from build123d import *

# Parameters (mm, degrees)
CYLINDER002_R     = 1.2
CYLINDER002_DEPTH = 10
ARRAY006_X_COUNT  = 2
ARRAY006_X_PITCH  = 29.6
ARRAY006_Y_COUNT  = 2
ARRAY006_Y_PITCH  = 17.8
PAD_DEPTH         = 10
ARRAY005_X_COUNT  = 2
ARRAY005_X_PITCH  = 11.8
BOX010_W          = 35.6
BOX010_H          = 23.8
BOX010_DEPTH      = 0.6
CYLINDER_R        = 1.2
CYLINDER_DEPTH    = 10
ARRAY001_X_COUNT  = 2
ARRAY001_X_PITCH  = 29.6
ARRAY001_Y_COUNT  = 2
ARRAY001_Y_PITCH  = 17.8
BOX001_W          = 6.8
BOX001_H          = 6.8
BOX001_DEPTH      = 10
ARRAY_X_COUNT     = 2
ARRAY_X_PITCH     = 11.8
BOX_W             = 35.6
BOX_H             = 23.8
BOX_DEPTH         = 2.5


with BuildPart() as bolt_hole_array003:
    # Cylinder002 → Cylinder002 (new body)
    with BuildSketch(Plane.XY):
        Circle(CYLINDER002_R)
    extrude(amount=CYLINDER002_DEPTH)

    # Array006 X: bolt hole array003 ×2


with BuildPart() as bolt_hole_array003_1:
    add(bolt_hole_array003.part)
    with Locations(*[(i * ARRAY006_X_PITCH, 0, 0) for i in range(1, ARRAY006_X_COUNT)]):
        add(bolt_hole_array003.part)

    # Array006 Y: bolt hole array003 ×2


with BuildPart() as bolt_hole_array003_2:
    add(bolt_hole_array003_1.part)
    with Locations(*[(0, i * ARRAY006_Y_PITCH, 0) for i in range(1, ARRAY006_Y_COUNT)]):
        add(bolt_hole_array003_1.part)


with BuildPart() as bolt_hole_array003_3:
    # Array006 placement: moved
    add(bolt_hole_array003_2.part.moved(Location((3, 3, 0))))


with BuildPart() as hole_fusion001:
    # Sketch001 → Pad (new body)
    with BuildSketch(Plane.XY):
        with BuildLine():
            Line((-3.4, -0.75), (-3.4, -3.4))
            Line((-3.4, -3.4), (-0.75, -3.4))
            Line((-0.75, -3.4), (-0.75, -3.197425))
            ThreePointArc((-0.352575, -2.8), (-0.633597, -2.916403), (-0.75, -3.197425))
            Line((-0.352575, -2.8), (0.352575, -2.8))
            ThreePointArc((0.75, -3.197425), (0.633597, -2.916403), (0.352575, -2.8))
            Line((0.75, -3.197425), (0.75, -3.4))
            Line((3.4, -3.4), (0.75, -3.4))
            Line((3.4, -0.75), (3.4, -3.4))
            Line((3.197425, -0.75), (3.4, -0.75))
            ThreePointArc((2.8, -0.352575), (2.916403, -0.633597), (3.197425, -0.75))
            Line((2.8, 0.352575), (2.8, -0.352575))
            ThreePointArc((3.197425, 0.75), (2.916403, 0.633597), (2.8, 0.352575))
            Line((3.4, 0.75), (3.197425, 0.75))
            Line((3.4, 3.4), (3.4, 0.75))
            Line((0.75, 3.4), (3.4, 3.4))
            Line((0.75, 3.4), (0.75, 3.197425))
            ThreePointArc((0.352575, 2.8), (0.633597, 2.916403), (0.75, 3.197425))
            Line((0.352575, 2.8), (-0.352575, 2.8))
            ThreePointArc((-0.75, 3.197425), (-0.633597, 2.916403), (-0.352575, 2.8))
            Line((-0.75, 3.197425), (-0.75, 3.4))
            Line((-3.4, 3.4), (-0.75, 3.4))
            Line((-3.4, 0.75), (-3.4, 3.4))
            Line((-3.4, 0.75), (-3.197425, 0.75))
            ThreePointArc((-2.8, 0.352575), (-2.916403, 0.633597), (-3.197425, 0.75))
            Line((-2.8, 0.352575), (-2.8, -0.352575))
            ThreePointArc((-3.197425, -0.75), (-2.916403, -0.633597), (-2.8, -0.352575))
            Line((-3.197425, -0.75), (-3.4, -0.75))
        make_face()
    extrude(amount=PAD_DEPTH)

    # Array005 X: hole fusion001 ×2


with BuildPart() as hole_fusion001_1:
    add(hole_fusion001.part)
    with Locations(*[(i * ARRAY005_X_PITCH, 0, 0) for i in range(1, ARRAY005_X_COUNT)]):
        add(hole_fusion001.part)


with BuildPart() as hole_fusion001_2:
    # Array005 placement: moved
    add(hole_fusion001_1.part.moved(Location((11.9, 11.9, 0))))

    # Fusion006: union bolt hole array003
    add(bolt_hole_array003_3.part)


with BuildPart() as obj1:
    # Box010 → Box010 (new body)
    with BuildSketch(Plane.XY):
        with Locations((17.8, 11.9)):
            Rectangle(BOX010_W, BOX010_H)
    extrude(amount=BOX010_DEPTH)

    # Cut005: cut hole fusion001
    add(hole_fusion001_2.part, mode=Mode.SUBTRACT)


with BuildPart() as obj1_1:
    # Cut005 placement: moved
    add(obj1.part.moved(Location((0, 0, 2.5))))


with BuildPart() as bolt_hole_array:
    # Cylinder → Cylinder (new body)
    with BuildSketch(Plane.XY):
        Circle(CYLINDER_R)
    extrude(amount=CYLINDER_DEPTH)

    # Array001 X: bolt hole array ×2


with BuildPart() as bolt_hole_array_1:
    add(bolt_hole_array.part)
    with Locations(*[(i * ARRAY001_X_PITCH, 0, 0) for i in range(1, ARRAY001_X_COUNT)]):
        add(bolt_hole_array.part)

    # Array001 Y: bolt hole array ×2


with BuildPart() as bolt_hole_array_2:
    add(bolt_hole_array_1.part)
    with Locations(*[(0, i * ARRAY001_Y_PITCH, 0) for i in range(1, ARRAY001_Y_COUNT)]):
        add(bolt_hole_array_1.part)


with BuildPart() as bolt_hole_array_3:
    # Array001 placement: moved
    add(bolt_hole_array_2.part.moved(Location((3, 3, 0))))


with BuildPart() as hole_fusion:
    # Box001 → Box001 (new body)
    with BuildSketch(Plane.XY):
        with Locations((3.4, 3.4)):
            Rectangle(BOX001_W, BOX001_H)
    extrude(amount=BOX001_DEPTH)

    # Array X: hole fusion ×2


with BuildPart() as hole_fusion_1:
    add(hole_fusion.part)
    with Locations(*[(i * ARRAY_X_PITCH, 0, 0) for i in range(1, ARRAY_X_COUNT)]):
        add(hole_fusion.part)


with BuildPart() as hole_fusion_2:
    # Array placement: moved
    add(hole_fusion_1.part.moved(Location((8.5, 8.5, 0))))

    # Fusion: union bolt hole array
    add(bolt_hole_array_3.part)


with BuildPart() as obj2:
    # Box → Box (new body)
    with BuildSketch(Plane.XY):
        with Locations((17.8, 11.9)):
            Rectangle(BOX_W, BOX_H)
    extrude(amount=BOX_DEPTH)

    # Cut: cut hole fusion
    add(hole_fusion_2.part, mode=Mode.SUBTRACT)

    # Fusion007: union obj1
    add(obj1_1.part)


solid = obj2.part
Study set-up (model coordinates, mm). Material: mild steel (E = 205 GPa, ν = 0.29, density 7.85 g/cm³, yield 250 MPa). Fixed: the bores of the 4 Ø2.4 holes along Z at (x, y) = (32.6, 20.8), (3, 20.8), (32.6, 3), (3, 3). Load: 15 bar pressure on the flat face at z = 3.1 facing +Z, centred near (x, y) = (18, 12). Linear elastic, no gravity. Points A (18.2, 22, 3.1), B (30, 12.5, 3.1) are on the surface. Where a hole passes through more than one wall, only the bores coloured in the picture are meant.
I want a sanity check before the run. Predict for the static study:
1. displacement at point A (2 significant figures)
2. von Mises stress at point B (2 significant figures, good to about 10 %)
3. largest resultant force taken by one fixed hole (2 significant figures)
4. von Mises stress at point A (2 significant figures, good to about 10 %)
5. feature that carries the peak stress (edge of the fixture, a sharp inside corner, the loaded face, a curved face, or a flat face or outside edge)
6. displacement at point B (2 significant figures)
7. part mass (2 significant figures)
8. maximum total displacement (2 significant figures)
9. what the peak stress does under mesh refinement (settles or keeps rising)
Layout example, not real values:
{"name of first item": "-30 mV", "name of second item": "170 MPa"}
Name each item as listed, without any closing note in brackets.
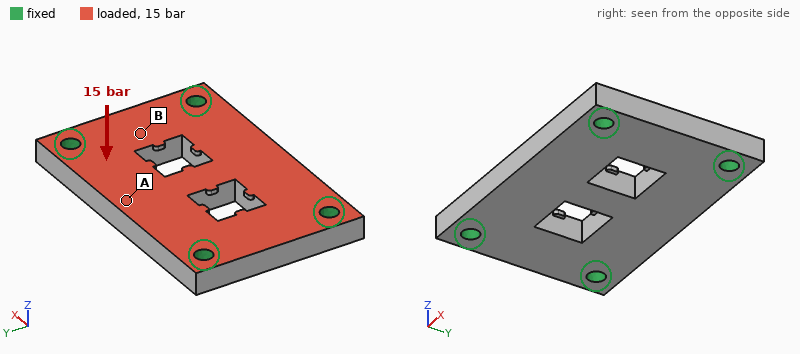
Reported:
{"displacement at point A": "6.9 µm", "von Mises stress at point B": "17 MPa", "largest resultant force taken by one fixed hole": "280 N", "von Mises stress at point A": "37 MPa", "feature that carries the peak stress": "edge of the fixture", "displacement at point B": "2.6 µm", "part mass": "18 g", "maximum total displacement": "8.6 µm", "what the peak stress does under mesh refinement": "keeps rising"}
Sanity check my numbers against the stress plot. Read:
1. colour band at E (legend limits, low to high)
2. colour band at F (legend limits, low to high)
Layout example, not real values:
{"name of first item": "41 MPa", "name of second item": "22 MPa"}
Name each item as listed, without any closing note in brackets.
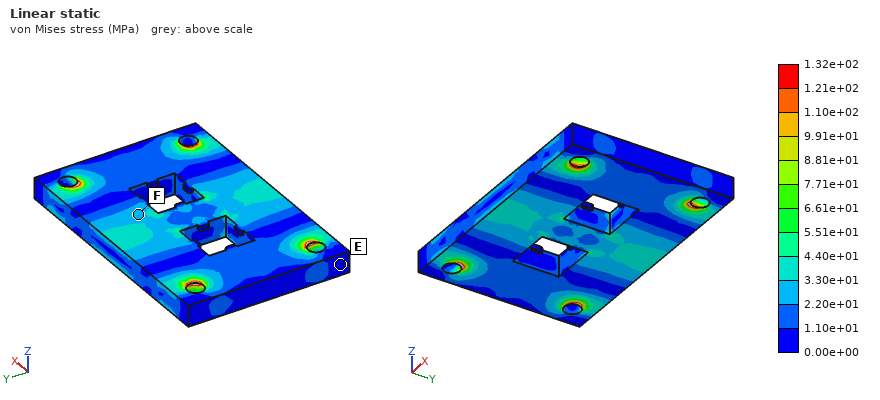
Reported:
{"colour band at E": "0.00e+00 to 1.10e+01 MPa", "colour band at F": "2.20e+01 to 3.30e+01 MPa"}
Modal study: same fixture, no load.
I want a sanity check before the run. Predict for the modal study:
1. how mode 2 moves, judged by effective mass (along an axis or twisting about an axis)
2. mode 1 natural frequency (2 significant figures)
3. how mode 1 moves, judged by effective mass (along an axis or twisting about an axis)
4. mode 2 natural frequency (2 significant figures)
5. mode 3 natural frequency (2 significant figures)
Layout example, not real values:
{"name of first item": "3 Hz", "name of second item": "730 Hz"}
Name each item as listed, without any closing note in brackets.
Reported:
{"how mode 2 moves, judged by effective mass": "twisting about X", "mode 1 natural frequency": "16 kHz", "how mode 1 moves, judged by effective mass": "along Z", "mode 2 natural frequency": "22 kHz", "mode 3 natural frequency": "35 kHz"}
